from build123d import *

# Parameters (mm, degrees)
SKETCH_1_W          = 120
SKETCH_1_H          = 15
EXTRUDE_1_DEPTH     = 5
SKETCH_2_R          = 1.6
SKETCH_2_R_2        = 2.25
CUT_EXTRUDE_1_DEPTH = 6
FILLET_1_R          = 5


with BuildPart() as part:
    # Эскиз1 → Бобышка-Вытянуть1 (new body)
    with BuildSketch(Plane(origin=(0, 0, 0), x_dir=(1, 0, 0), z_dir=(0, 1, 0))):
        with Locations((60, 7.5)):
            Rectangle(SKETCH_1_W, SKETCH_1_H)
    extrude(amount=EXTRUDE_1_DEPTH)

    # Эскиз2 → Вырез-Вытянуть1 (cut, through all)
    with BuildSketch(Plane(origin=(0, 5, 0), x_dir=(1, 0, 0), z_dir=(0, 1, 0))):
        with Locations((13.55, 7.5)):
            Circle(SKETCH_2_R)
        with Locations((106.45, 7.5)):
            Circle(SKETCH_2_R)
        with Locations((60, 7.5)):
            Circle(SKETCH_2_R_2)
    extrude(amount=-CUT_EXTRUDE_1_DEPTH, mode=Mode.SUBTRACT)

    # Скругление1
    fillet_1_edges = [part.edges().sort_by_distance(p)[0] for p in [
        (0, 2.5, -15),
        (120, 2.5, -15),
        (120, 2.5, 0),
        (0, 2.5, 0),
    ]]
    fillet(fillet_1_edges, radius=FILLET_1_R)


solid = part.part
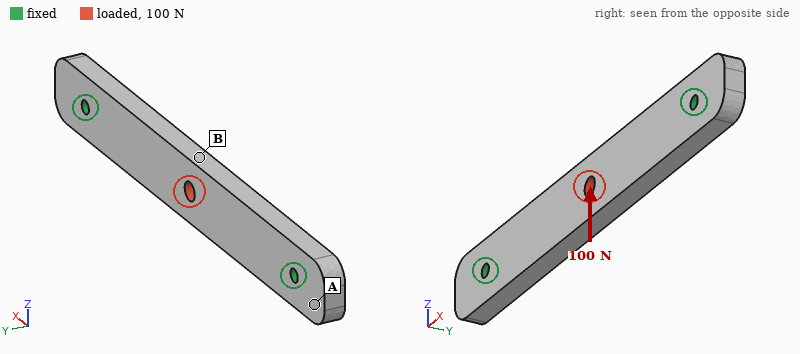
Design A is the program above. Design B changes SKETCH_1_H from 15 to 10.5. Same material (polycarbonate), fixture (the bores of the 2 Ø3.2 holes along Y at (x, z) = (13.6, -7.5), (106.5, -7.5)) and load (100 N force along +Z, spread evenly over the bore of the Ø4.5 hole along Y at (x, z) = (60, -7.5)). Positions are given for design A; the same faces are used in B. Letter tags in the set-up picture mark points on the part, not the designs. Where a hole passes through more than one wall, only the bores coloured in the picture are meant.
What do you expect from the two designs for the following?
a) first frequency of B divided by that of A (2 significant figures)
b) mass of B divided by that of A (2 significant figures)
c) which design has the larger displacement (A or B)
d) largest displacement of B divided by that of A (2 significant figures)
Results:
1.0
0.69
B
2.0
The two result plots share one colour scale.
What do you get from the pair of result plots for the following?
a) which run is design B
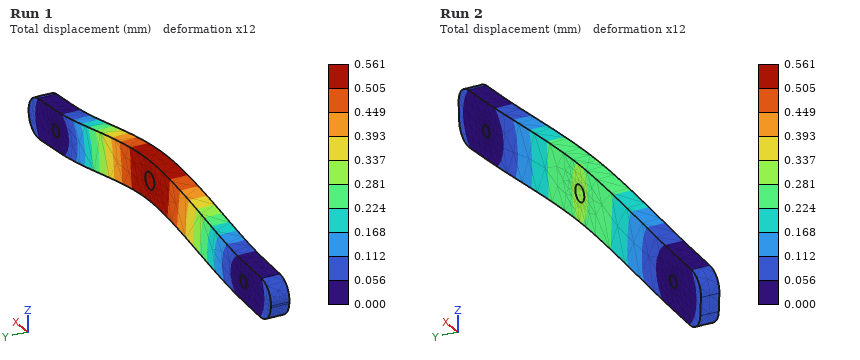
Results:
Run 1
